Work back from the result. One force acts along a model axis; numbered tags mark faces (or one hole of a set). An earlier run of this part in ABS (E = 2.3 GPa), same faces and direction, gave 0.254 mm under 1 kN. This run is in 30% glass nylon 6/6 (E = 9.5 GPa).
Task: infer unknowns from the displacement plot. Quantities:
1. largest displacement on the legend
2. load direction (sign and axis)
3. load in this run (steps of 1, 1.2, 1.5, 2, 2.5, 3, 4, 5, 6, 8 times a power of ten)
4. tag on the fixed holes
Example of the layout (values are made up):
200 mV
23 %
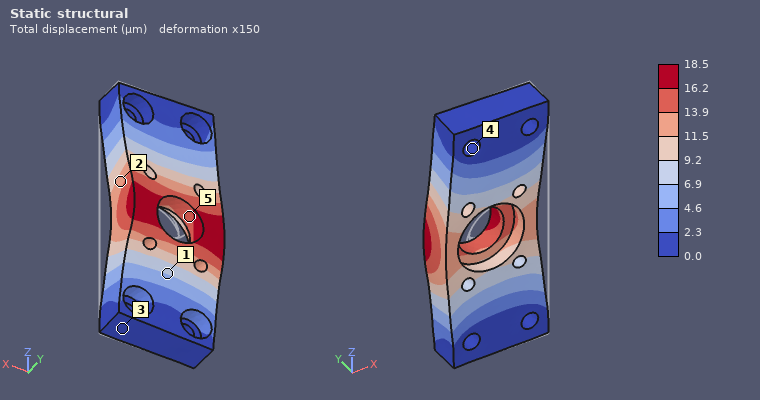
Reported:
18.5 µm
-X
300 N
4
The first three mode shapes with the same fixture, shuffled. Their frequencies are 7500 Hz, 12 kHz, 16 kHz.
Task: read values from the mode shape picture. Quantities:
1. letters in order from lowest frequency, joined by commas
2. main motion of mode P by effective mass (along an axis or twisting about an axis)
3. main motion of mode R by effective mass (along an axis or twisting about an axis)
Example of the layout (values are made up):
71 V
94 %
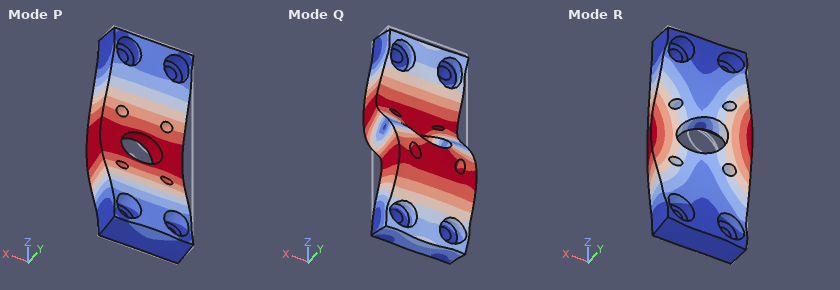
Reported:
P, R, Q
along Y
twisting about Z
